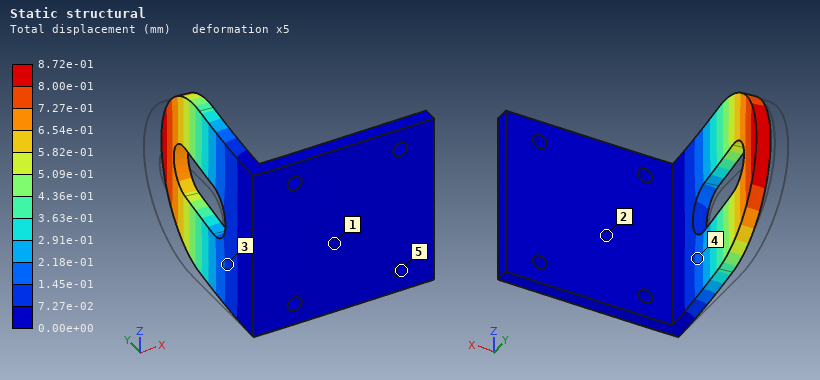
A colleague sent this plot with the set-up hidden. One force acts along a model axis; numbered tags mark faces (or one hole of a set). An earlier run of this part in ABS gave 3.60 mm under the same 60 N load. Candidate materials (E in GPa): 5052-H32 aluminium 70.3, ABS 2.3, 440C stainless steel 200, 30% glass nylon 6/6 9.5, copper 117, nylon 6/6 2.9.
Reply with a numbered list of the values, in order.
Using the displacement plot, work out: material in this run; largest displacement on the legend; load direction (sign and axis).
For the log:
1. 30% glass nylon 6/6
2. 8.72e-01 mm
3. +X
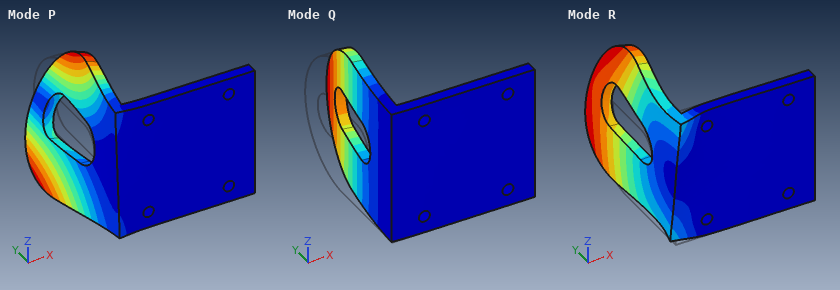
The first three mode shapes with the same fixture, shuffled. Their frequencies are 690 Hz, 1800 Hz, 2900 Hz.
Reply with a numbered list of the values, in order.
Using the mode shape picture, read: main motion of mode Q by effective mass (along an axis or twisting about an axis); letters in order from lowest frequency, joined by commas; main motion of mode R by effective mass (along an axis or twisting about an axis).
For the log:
1. along X
2. Q, P, R
3. along Z
